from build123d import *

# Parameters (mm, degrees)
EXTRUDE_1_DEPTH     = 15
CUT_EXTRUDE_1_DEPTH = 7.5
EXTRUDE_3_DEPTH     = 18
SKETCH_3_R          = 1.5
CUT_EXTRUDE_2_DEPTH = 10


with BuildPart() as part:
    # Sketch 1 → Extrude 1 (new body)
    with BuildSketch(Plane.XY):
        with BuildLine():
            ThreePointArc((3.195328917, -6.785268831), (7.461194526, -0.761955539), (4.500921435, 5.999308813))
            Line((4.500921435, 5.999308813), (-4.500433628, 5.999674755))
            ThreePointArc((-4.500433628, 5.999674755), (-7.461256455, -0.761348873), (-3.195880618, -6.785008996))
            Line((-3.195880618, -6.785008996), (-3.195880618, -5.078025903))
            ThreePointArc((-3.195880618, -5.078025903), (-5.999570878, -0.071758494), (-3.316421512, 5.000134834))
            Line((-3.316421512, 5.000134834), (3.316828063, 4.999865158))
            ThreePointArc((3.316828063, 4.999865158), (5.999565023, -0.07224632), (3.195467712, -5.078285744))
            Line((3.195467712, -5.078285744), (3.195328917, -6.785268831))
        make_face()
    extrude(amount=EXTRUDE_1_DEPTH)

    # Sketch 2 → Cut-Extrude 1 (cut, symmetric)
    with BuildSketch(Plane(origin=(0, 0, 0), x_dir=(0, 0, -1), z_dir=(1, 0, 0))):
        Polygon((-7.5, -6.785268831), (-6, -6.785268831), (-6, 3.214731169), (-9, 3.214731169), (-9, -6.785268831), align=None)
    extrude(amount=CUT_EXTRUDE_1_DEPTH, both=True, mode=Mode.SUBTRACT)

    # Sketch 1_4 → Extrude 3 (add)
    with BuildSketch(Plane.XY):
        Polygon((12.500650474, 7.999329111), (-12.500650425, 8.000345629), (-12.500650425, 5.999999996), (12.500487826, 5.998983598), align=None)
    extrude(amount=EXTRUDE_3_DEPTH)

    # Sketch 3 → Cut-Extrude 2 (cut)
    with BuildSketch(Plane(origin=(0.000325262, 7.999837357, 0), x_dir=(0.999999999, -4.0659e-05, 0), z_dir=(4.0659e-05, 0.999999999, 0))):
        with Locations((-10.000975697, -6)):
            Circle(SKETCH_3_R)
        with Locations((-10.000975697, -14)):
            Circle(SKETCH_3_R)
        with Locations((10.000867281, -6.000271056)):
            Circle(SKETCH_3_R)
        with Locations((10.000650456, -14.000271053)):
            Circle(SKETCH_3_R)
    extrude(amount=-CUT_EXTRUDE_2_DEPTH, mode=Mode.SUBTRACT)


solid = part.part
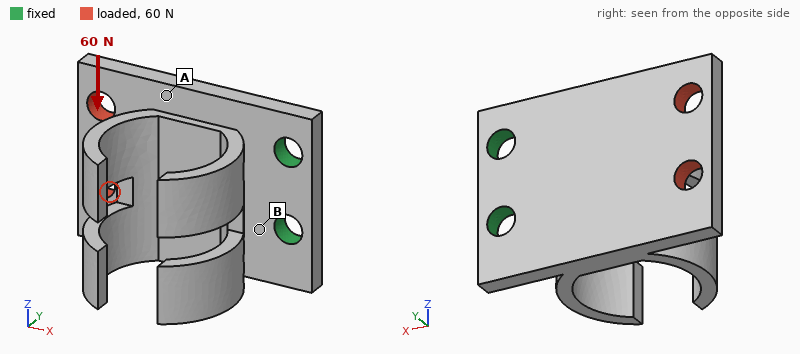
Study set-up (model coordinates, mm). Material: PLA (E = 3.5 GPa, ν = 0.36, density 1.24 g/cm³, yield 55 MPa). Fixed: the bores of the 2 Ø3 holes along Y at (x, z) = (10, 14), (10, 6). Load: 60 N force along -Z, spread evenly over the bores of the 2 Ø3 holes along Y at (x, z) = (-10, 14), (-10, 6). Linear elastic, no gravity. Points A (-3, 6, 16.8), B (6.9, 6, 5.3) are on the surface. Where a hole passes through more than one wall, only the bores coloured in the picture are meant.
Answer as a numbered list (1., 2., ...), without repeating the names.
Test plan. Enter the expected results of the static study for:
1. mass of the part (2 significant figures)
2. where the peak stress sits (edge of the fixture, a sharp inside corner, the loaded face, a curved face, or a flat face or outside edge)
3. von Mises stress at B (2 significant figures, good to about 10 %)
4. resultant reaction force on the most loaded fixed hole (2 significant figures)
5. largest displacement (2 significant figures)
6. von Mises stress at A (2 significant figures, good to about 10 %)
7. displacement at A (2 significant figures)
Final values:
1. 1.8 g
2. edge of the fixture
3. 10 MPa
4. 120 N
5. 0.13 mm
6. 2.8 MPa
7. 0.065 mm
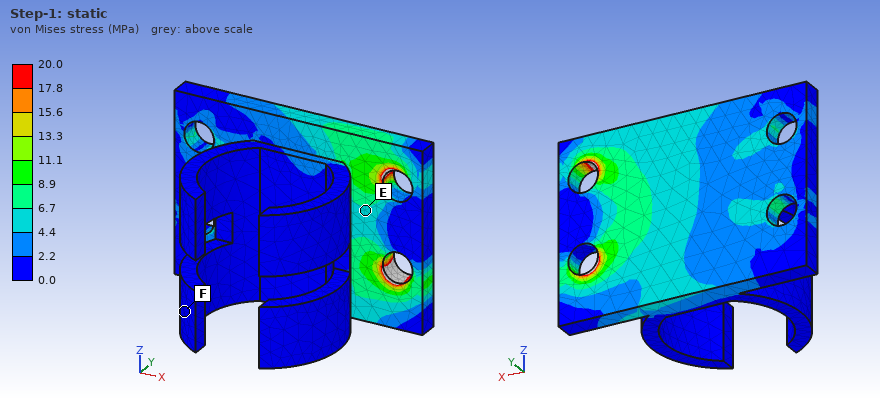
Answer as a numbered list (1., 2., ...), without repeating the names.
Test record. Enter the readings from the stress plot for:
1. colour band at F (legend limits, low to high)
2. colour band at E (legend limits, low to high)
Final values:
1. 0.0 to 2.2 MPa
2. 4.4 to 6.7 MPa
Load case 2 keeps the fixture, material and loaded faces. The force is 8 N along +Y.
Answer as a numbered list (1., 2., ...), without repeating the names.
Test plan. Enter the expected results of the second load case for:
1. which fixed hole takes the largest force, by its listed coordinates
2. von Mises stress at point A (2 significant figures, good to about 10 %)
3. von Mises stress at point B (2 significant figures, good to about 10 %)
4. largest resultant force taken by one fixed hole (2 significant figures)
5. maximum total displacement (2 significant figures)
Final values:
1. (10, 6)
2. 2.3 MPa
3. 12 MPa
4. 4.3 N
5. 0.41 mm
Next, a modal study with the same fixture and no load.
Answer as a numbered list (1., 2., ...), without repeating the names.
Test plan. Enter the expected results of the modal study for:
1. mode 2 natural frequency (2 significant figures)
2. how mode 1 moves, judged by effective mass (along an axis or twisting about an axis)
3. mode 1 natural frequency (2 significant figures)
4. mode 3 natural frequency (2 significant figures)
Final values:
1. 2100 Hz
2. along Y
3. 950 Hz
4. 2300 Hz
